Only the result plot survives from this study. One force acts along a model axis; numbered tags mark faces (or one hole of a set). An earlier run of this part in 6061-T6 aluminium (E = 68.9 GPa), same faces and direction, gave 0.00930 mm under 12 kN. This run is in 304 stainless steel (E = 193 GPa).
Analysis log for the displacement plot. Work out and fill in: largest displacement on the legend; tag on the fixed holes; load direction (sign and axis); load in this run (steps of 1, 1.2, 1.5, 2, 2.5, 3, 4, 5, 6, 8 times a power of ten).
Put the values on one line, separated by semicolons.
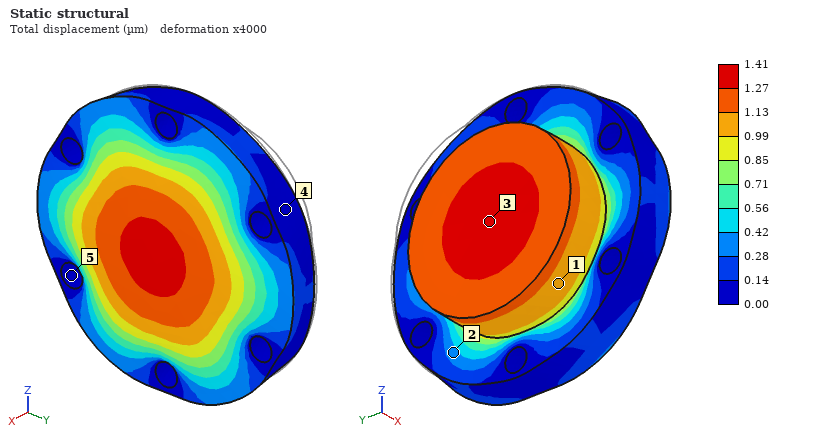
1.41 µm; 5; +X; 5 kN
